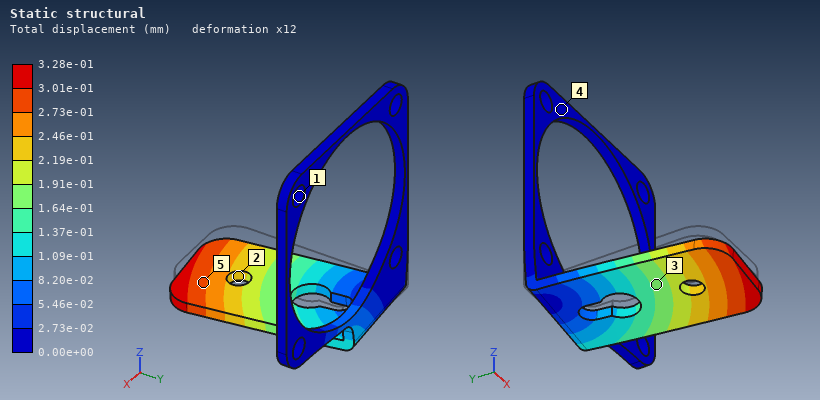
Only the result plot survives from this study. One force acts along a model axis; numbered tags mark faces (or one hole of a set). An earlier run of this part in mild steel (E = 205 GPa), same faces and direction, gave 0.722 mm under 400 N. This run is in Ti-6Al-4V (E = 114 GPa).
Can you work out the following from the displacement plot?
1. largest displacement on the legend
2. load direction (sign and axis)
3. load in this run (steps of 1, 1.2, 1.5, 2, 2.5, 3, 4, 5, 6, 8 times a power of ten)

3.28e-01 mm
+X
100 N
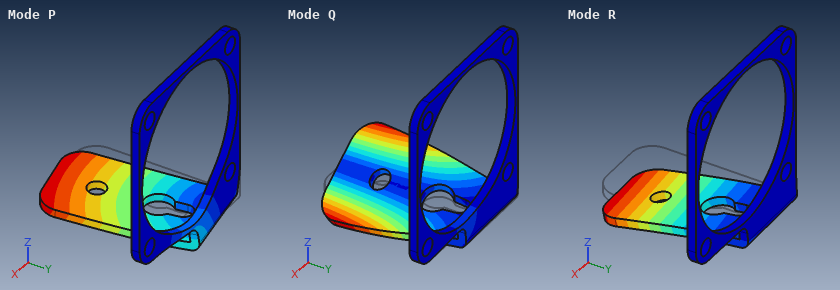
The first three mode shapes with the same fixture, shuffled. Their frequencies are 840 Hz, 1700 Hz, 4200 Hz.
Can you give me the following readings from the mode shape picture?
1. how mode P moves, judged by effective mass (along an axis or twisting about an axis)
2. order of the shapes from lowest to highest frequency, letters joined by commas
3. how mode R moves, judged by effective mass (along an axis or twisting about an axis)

along X
R, P, Q
along Z
